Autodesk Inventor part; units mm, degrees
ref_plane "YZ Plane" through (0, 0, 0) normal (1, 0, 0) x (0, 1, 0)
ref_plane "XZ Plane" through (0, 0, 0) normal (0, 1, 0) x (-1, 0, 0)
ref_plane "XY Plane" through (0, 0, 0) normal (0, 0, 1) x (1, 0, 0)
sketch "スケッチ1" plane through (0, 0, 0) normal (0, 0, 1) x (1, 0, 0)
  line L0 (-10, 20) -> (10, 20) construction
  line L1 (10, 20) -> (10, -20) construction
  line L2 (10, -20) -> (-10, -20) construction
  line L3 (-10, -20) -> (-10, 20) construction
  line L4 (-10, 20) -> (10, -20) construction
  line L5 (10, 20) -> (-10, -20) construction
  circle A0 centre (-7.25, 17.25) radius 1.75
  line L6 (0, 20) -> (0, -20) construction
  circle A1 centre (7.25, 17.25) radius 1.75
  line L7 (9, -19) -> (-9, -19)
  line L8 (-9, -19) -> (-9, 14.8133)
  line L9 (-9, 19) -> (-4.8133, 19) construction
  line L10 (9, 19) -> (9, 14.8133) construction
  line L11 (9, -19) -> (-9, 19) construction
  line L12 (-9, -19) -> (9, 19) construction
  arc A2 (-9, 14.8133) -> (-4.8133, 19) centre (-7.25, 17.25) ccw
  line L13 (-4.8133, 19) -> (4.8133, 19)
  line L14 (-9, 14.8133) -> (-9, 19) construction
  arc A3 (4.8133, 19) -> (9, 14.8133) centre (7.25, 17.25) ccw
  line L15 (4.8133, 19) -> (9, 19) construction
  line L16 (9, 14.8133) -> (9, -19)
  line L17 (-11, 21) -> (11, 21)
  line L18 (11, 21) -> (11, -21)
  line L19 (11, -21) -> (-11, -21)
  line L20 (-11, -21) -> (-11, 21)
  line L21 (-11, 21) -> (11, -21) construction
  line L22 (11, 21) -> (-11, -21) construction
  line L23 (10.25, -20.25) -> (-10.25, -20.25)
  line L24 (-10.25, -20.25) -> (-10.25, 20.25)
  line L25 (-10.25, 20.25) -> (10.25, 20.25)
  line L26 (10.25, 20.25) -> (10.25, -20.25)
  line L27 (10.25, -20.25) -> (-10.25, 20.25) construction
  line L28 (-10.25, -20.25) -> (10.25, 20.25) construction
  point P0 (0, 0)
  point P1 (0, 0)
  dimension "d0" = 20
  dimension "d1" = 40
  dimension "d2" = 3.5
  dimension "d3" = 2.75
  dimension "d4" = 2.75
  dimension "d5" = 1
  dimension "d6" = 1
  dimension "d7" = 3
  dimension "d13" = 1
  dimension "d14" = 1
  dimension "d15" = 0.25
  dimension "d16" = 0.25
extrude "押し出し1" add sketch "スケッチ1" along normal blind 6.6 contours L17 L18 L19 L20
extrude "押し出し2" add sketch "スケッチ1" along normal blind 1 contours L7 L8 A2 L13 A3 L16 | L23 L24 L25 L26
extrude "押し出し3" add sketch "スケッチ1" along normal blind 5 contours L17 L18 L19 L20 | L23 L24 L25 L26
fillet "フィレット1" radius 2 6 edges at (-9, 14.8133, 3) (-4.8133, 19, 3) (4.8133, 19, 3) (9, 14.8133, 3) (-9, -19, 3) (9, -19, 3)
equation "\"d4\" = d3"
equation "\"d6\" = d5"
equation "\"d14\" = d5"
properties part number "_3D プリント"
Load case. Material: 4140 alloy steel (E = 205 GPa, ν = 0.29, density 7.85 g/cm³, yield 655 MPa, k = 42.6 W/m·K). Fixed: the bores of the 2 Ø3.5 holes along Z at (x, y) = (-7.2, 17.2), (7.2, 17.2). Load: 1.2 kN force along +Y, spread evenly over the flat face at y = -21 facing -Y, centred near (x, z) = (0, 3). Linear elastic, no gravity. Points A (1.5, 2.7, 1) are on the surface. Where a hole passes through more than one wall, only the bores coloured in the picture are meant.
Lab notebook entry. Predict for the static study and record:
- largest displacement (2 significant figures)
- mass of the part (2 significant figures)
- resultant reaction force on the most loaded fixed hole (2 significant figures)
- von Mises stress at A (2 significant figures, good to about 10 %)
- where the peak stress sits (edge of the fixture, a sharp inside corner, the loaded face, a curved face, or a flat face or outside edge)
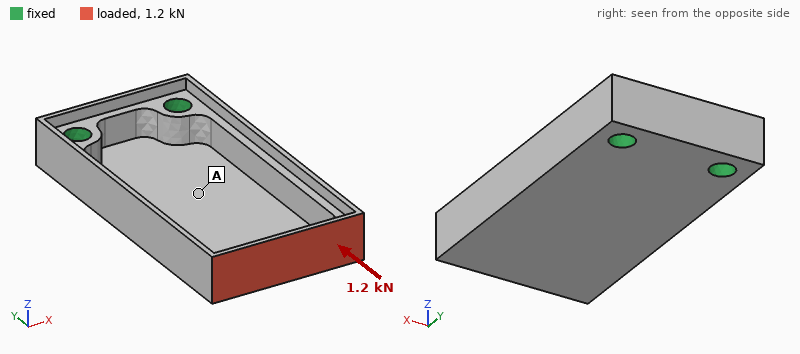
82 µm
17 g
600 N
18 MPa
a curved face
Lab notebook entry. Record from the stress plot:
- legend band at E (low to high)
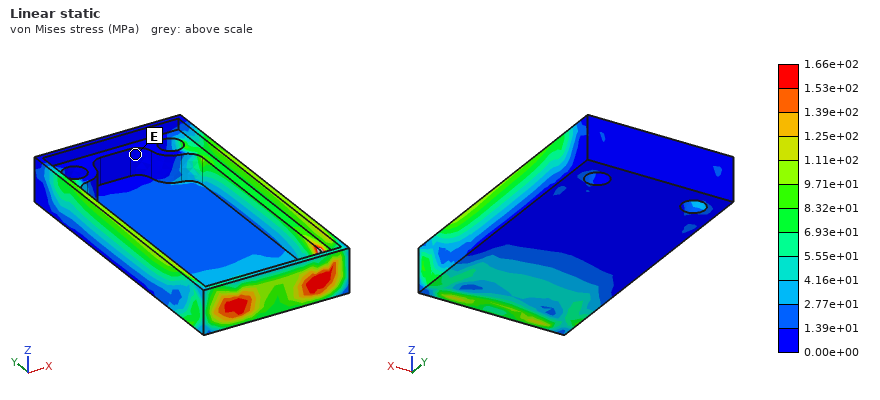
0.00e+00 to 1.39e+01 MPa
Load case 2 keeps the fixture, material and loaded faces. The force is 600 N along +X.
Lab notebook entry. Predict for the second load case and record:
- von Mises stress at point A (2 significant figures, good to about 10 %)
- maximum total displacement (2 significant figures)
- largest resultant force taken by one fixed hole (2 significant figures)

110 MPa
0.19 mm
1.3 kN
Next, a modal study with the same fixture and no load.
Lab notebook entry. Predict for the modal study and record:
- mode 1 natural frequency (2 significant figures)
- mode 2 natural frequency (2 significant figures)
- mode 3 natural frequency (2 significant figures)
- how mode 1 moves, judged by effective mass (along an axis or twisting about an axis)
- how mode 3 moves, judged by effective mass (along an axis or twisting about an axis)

2700 Hz
3900 Hz
10 kHz
along Z
along X
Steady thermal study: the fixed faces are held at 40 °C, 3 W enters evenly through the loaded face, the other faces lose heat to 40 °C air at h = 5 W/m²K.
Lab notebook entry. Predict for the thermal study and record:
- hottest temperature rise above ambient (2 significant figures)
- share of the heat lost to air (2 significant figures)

62 K
13 %
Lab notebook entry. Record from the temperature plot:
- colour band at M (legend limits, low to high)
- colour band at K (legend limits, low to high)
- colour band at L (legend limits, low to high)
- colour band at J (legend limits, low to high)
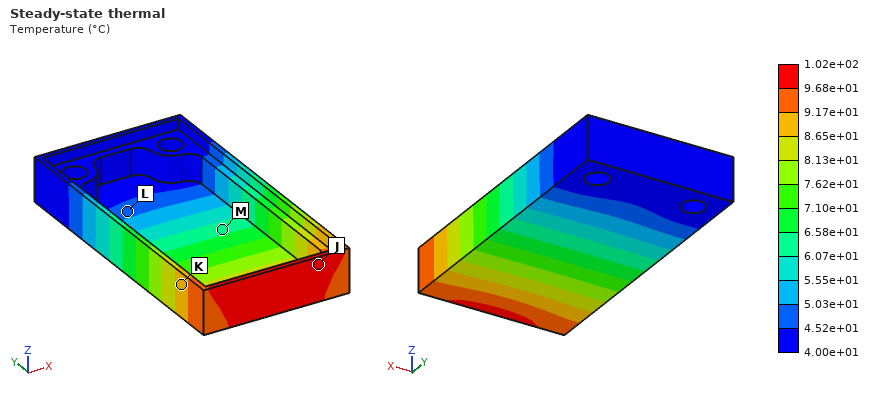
6.07e+01 to 6.58e+01 °C
8.65e+01 to 9.17e+01 °C
4.52e+01 to 5.03e+01 °C
9.68e+01 to 1.02e+02 °C
